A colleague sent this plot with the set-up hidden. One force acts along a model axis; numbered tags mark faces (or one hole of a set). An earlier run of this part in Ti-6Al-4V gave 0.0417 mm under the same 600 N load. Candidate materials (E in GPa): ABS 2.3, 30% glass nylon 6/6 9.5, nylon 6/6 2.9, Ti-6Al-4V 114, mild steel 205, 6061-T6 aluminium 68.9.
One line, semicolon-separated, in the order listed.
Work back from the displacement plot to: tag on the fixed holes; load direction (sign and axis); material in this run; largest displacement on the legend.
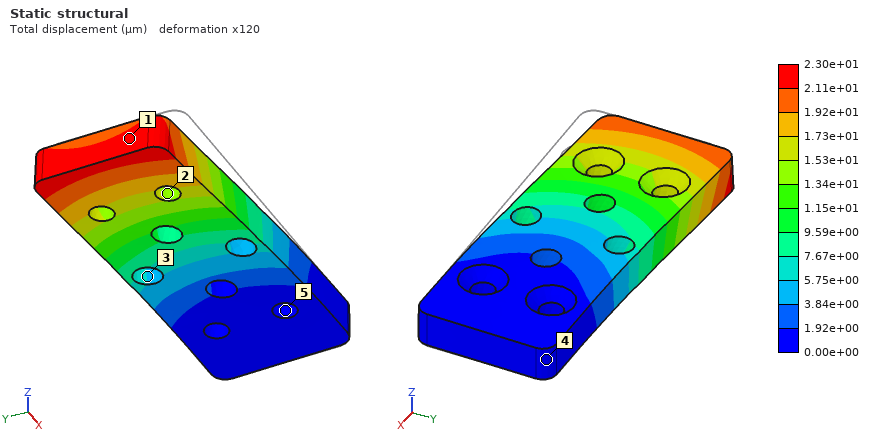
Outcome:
5; +Y; mild steel; 2.30e+01 µm
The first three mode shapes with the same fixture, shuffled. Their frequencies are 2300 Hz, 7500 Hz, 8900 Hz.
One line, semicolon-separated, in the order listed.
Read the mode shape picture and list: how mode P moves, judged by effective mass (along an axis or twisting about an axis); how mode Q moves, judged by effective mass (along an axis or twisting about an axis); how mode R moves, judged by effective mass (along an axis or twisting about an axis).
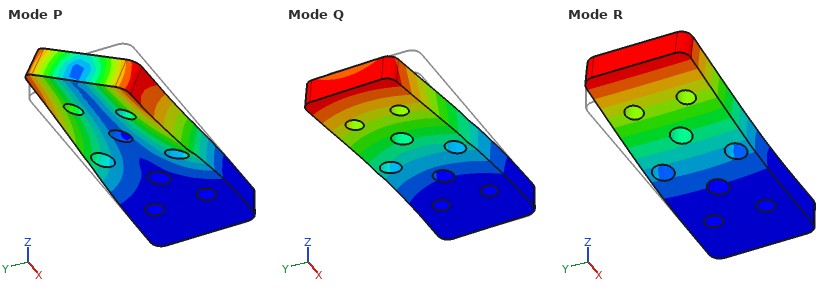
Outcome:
twisting about X; along Y; along Z
